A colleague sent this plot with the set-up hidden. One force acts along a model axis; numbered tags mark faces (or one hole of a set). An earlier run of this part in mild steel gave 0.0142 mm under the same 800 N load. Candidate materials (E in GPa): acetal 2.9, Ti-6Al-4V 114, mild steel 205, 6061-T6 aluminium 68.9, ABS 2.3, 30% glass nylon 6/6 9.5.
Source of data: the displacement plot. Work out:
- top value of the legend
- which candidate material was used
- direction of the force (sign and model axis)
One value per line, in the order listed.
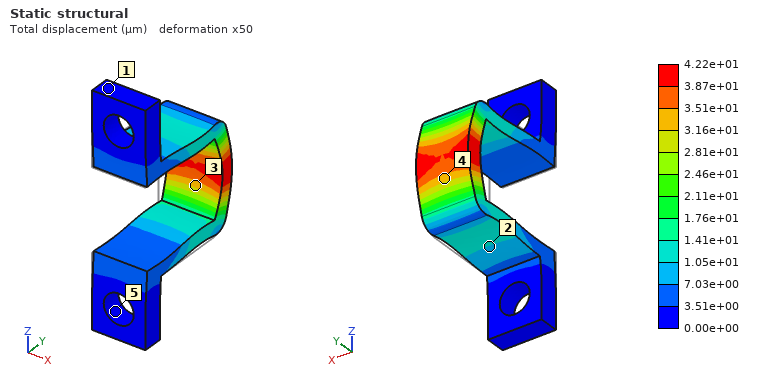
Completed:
4.22e+01 µm
6061-T6 aluminium
+Y
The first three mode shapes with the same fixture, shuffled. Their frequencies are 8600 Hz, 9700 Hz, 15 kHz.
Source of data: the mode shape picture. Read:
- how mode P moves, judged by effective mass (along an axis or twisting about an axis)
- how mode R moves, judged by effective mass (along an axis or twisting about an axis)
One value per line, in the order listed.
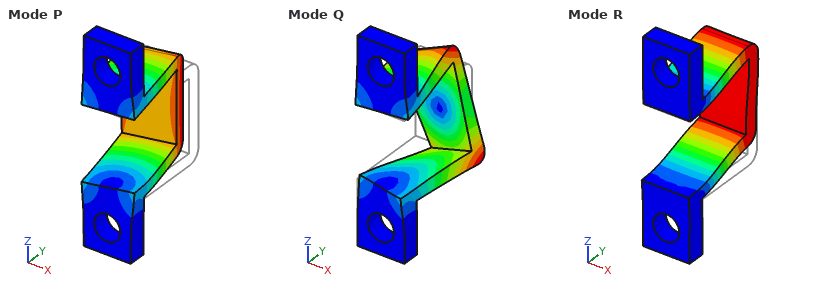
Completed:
along X
along Z
